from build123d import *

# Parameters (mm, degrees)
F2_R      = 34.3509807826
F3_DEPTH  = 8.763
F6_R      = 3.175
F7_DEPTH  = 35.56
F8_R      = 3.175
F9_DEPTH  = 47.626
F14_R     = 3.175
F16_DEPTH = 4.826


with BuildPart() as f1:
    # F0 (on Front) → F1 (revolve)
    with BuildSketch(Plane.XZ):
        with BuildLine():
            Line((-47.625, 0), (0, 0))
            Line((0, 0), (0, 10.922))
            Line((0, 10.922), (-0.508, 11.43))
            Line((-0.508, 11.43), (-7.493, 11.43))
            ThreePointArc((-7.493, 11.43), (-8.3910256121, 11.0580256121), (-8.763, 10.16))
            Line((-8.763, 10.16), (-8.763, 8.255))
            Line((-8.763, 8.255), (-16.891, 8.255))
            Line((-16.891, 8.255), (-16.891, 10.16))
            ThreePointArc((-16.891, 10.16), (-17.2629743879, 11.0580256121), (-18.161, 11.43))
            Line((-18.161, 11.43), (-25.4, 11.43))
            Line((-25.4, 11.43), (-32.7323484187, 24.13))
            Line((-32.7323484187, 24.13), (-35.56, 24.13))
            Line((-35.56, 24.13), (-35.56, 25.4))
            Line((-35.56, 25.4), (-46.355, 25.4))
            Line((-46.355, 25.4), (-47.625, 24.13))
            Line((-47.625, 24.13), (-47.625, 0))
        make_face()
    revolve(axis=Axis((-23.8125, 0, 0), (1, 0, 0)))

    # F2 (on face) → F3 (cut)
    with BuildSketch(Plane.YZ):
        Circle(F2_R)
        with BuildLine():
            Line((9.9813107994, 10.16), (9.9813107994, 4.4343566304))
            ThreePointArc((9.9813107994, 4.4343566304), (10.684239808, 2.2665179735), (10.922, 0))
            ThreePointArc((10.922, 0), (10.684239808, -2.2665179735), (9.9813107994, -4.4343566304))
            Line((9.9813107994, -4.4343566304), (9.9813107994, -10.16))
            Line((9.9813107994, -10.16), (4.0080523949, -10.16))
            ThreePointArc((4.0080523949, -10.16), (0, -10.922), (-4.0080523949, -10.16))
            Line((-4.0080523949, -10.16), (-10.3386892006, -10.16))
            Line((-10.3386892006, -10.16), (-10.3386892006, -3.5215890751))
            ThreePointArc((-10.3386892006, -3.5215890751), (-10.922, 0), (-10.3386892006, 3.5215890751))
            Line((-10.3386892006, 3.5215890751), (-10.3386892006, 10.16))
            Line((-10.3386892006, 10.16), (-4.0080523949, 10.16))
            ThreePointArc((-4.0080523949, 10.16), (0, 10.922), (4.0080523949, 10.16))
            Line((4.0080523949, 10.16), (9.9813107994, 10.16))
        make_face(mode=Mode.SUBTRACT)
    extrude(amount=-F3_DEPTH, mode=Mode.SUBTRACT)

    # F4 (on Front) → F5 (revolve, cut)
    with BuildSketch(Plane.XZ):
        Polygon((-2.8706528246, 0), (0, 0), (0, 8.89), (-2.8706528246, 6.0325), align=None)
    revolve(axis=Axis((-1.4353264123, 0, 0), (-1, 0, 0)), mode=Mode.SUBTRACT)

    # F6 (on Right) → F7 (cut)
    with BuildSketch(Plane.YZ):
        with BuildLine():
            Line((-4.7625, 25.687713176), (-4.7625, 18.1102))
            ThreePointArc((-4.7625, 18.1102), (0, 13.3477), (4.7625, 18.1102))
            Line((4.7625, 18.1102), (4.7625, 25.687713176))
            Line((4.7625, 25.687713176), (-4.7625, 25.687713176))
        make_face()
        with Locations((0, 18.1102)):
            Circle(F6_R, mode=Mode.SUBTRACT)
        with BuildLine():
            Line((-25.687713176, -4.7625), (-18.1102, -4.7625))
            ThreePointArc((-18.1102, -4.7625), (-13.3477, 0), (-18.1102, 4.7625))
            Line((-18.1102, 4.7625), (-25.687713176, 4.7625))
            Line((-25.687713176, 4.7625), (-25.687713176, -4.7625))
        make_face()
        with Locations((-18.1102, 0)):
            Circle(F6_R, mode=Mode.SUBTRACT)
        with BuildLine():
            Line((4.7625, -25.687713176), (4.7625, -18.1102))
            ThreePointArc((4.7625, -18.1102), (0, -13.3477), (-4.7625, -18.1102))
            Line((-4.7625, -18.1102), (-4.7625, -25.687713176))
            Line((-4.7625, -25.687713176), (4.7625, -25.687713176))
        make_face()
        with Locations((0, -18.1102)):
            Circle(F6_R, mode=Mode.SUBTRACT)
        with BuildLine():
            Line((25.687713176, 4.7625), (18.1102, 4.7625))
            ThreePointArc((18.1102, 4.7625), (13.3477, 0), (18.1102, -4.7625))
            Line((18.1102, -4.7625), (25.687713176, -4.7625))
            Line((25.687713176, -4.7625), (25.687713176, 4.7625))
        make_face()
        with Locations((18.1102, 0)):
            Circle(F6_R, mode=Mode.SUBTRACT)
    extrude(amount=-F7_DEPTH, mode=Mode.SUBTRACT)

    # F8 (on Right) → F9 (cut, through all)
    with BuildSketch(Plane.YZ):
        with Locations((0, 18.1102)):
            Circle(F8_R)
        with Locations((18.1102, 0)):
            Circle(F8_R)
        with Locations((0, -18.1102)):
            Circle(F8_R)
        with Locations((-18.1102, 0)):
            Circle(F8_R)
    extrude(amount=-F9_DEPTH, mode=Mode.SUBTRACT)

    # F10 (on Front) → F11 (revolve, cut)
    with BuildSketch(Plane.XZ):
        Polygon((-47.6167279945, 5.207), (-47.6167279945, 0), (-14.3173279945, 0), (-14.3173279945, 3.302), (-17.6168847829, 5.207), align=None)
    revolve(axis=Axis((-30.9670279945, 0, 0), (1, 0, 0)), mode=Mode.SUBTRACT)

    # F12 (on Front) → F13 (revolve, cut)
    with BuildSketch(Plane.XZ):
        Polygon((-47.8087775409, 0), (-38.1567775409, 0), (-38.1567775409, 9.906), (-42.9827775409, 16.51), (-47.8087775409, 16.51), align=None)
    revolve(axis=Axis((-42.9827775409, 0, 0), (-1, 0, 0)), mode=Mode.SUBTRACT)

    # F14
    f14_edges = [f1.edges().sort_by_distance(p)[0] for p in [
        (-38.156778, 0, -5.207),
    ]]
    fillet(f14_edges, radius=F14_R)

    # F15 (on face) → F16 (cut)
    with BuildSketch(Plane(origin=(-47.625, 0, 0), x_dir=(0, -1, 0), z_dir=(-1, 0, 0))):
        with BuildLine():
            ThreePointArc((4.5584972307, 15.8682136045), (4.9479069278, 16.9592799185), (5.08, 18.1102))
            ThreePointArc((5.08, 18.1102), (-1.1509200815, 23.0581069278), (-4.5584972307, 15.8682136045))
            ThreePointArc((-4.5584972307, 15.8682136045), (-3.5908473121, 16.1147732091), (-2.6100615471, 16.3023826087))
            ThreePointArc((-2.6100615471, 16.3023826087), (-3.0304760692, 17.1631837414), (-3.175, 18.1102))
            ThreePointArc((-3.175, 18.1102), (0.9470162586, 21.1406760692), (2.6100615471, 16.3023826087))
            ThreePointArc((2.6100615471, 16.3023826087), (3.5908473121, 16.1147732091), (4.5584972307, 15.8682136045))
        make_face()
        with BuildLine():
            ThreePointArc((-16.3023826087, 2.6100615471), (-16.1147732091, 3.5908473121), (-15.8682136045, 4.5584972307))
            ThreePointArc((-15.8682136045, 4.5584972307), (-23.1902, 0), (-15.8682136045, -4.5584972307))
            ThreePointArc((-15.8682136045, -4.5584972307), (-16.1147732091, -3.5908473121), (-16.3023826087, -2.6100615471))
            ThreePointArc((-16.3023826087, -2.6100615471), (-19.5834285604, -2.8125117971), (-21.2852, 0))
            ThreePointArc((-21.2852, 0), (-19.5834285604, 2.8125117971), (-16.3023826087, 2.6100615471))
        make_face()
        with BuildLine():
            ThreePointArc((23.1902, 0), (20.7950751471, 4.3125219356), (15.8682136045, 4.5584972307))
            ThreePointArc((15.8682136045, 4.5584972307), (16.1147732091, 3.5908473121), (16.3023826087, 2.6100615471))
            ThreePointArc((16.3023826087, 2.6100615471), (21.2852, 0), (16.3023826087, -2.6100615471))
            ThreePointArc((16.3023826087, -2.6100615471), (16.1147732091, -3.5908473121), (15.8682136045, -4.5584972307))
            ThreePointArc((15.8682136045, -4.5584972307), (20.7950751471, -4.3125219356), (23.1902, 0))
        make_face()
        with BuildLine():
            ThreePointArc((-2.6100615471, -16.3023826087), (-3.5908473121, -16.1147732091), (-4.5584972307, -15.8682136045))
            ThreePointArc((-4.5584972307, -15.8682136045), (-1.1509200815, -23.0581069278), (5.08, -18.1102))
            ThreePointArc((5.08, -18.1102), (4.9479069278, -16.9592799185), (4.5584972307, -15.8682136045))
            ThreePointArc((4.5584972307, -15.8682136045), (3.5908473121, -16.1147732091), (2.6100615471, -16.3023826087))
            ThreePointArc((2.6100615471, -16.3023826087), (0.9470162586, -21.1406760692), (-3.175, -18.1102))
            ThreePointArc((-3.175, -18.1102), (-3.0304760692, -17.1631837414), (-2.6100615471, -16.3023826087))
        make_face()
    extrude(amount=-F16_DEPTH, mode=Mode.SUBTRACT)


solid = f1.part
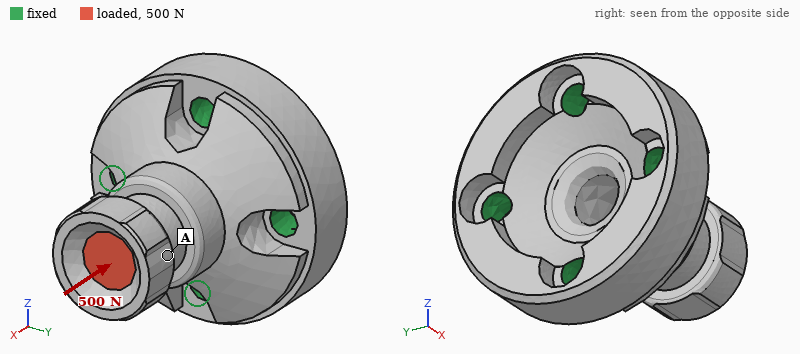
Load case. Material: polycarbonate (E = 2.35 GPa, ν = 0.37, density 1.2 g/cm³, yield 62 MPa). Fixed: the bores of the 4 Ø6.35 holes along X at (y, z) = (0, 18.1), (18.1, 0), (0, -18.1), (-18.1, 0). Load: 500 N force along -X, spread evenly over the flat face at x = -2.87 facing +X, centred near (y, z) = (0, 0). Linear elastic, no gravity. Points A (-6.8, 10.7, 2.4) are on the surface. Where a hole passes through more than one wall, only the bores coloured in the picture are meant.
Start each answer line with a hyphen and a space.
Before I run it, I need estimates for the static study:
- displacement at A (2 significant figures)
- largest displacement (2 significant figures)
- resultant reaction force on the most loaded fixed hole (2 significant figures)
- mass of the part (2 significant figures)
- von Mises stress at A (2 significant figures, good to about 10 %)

- 27 µm
- 38 µm
- 140 N
- 39 g
- 0.62 MPa
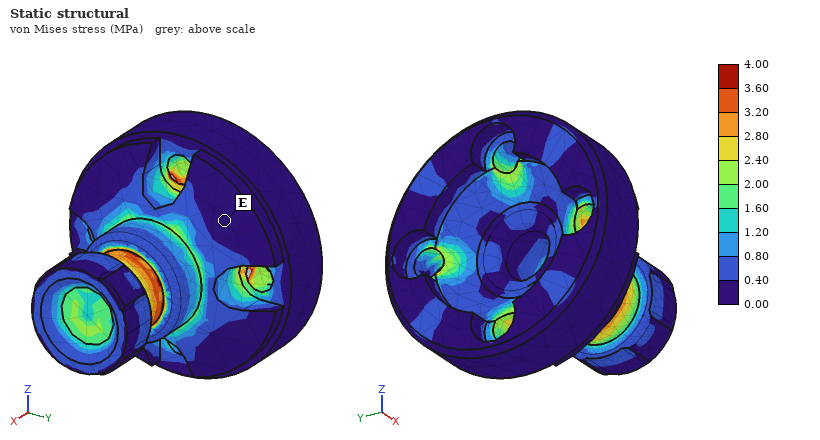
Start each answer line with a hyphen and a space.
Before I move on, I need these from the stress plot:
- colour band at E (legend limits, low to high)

- 0.00 to 0.40 MPa
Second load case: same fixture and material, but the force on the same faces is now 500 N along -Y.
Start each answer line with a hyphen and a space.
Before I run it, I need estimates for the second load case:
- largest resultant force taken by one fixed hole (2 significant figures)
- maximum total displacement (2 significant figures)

- 510 N
- 0.34 mm
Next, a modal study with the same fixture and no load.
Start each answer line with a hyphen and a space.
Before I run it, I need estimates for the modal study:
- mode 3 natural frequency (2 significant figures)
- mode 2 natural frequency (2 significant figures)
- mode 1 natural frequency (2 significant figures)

- 6100 Hz
- 3400 Hz
- 3400 Hz
